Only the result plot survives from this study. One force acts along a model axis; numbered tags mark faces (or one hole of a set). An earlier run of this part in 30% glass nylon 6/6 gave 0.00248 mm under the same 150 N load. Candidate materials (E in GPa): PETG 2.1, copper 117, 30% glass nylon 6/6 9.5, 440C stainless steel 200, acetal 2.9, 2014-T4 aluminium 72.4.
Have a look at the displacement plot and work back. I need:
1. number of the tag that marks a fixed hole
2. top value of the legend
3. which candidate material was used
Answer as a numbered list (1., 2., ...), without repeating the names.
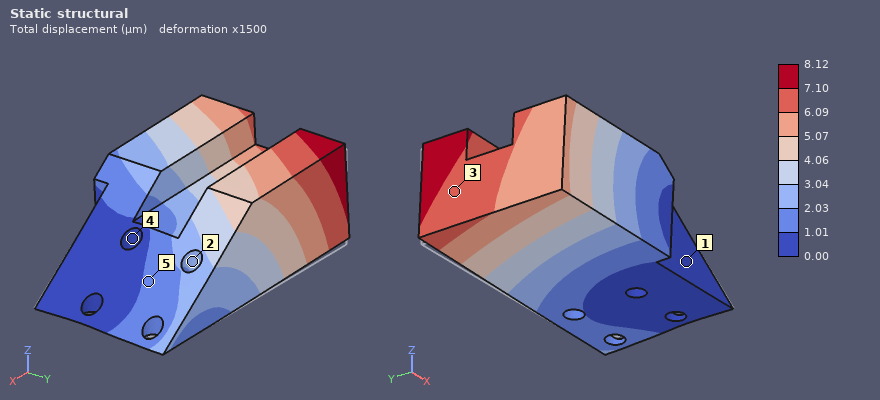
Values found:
1. 4
2. 8.12 µm
3. acetal
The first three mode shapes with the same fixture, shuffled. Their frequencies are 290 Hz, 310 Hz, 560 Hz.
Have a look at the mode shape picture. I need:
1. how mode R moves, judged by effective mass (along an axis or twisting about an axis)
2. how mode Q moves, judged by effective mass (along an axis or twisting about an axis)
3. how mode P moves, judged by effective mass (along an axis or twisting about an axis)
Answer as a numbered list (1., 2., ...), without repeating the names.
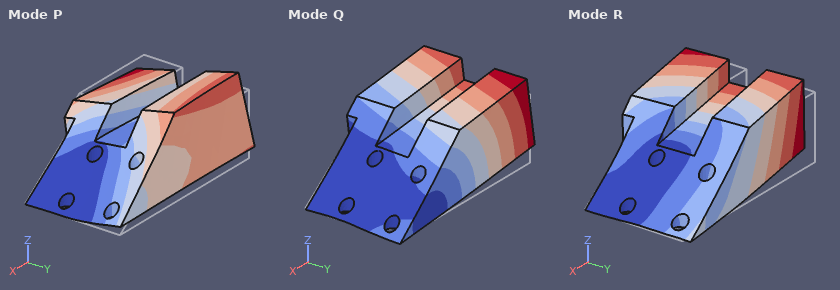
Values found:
1. along Y
2. along Z
3. twisting about X
